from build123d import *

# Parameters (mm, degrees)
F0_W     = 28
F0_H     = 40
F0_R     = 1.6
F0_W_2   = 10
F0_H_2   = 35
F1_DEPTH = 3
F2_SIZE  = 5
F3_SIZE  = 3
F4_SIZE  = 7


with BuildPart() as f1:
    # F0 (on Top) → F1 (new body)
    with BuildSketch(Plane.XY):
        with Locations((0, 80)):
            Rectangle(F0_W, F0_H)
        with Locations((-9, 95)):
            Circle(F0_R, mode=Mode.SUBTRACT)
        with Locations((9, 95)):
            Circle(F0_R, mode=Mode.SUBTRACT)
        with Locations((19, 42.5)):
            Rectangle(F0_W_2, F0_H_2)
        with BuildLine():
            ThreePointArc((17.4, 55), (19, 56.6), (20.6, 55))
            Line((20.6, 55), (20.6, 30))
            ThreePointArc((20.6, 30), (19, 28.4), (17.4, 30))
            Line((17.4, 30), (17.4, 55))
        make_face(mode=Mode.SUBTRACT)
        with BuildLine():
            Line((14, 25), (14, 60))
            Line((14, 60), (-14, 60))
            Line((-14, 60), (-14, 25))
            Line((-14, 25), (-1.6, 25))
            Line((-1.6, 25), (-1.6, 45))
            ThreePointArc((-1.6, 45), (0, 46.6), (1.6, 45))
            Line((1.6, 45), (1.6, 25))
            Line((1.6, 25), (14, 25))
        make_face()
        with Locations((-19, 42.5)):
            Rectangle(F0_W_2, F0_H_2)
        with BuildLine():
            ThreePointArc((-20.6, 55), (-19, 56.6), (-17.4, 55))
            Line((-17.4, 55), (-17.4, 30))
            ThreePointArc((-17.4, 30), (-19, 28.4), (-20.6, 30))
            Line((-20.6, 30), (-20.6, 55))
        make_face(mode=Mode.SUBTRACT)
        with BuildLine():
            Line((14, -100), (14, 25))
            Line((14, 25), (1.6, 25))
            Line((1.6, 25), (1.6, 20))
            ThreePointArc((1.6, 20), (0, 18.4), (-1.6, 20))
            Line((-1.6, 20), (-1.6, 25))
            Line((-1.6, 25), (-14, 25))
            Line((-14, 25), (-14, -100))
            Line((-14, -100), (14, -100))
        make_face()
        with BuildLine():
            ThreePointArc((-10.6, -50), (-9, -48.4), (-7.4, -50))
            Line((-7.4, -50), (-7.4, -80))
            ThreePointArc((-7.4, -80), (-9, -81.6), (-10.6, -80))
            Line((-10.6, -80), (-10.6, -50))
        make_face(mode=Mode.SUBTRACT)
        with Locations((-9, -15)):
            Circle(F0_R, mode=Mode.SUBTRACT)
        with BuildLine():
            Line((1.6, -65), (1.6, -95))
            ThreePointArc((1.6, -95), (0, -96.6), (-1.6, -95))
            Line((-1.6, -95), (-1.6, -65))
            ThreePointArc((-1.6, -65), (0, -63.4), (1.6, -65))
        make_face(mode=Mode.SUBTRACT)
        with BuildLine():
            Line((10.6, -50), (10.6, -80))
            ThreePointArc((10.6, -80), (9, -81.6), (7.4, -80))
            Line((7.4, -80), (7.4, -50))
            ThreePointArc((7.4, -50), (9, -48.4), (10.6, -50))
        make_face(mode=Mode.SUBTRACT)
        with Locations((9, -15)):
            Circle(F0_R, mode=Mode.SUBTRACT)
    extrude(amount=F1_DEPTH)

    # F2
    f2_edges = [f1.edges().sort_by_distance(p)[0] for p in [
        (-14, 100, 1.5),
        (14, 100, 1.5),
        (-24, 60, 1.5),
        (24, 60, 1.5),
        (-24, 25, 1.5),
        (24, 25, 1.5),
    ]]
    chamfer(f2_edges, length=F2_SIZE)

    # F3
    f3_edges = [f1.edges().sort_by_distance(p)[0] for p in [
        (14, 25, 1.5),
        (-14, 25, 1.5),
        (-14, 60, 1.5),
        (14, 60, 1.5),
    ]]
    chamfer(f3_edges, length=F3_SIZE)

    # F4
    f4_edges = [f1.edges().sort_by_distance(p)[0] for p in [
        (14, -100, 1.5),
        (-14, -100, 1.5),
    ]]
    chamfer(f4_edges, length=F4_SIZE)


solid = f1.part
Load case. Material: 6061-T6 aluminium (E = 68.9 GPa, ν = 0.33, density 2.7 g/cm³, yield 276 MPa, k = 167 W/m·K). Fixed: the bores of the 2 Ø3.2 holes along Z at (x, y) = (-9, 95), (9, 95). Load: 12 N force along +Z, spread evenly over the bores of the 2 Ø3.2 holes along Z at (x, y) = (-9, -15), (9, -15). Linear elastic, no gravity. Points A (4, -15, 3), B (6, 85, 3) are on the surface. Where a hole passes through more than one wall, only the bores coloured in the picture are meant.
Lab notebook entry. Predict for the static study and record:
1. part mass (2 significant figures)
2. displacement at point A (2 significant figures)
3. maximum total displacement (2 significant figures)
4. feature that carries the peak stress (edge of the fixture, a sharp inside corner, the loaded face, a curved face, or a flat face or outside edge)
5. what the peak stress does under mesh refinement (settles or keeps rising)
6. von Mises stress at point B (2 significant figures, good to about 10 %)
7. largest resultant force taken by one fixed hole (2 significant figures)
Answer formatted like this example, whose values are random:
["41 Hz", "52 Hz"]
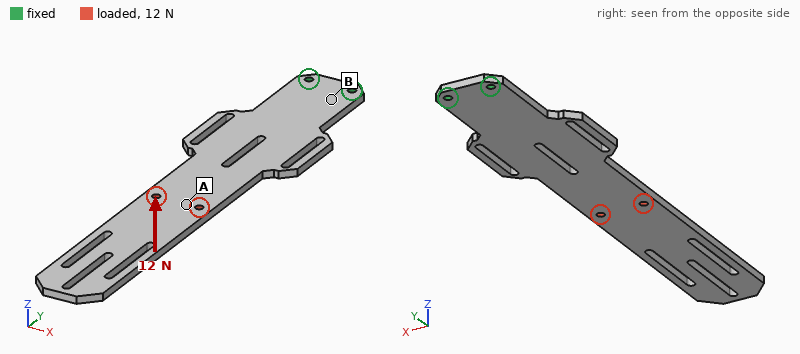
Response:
["45 g", "1.1 mm", "2.5 mm", "edge of the fixture", "keeps rising", "27 MPa", "6.0 N"]
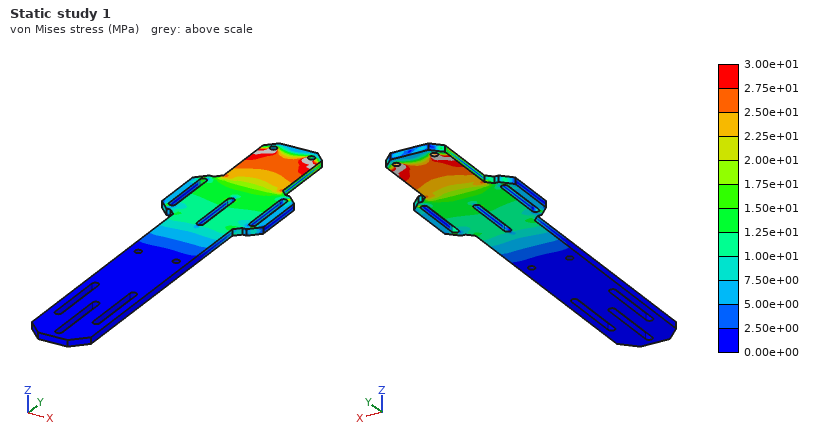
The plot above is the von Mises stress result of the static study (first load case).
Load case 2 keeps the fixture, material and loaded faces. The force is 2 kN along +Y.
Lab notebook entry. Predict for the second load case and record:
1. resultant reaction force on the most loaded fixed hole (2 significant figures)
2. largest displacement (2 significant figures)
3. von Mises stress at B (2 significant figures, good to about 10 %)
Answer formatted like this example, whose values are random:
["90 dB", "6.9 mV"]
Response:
["1.0 kN", "40 µm", "25 MPa"]
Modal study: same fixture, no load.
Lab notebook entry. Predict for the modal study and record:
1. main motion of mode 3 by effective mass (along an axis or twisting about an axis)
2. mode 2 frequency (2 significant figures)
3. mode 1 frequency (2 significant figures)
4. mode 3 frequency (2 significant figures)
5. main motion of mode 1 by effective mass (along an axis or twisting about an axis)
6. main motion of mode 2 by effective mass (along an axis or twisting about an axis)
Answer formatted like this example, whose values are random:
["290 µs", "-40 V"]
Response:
["along X", "400 Hz", "73 Hz", "680 Hz", "along Z", "along Z"]
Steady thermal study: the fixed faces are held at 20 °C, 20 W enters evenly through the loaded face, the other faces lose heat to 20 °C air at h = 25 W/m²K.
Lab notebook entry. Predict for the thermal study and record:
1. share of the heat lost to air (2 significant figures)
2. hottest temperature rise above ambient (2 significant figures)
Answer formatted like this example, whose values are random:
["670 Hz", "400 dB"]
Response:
["65 %", "70 K"]
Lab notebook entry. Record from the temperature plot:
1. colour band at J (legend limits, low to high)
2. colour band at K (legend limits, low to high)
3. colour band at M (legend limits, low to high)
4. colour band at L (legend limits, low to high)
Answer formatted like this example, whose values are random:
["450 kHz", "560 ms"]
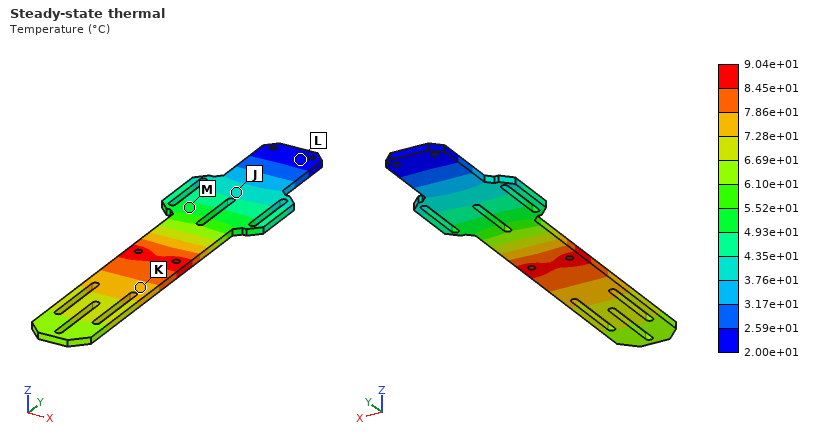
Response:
["3.76e+01 to 4.35e+01 °C", "7.28e+01 to 7.86e+01 °C", "4.93e+01 to 5.52e+01 °C", "2.00e+01 to 2.59e+01 °C"]
